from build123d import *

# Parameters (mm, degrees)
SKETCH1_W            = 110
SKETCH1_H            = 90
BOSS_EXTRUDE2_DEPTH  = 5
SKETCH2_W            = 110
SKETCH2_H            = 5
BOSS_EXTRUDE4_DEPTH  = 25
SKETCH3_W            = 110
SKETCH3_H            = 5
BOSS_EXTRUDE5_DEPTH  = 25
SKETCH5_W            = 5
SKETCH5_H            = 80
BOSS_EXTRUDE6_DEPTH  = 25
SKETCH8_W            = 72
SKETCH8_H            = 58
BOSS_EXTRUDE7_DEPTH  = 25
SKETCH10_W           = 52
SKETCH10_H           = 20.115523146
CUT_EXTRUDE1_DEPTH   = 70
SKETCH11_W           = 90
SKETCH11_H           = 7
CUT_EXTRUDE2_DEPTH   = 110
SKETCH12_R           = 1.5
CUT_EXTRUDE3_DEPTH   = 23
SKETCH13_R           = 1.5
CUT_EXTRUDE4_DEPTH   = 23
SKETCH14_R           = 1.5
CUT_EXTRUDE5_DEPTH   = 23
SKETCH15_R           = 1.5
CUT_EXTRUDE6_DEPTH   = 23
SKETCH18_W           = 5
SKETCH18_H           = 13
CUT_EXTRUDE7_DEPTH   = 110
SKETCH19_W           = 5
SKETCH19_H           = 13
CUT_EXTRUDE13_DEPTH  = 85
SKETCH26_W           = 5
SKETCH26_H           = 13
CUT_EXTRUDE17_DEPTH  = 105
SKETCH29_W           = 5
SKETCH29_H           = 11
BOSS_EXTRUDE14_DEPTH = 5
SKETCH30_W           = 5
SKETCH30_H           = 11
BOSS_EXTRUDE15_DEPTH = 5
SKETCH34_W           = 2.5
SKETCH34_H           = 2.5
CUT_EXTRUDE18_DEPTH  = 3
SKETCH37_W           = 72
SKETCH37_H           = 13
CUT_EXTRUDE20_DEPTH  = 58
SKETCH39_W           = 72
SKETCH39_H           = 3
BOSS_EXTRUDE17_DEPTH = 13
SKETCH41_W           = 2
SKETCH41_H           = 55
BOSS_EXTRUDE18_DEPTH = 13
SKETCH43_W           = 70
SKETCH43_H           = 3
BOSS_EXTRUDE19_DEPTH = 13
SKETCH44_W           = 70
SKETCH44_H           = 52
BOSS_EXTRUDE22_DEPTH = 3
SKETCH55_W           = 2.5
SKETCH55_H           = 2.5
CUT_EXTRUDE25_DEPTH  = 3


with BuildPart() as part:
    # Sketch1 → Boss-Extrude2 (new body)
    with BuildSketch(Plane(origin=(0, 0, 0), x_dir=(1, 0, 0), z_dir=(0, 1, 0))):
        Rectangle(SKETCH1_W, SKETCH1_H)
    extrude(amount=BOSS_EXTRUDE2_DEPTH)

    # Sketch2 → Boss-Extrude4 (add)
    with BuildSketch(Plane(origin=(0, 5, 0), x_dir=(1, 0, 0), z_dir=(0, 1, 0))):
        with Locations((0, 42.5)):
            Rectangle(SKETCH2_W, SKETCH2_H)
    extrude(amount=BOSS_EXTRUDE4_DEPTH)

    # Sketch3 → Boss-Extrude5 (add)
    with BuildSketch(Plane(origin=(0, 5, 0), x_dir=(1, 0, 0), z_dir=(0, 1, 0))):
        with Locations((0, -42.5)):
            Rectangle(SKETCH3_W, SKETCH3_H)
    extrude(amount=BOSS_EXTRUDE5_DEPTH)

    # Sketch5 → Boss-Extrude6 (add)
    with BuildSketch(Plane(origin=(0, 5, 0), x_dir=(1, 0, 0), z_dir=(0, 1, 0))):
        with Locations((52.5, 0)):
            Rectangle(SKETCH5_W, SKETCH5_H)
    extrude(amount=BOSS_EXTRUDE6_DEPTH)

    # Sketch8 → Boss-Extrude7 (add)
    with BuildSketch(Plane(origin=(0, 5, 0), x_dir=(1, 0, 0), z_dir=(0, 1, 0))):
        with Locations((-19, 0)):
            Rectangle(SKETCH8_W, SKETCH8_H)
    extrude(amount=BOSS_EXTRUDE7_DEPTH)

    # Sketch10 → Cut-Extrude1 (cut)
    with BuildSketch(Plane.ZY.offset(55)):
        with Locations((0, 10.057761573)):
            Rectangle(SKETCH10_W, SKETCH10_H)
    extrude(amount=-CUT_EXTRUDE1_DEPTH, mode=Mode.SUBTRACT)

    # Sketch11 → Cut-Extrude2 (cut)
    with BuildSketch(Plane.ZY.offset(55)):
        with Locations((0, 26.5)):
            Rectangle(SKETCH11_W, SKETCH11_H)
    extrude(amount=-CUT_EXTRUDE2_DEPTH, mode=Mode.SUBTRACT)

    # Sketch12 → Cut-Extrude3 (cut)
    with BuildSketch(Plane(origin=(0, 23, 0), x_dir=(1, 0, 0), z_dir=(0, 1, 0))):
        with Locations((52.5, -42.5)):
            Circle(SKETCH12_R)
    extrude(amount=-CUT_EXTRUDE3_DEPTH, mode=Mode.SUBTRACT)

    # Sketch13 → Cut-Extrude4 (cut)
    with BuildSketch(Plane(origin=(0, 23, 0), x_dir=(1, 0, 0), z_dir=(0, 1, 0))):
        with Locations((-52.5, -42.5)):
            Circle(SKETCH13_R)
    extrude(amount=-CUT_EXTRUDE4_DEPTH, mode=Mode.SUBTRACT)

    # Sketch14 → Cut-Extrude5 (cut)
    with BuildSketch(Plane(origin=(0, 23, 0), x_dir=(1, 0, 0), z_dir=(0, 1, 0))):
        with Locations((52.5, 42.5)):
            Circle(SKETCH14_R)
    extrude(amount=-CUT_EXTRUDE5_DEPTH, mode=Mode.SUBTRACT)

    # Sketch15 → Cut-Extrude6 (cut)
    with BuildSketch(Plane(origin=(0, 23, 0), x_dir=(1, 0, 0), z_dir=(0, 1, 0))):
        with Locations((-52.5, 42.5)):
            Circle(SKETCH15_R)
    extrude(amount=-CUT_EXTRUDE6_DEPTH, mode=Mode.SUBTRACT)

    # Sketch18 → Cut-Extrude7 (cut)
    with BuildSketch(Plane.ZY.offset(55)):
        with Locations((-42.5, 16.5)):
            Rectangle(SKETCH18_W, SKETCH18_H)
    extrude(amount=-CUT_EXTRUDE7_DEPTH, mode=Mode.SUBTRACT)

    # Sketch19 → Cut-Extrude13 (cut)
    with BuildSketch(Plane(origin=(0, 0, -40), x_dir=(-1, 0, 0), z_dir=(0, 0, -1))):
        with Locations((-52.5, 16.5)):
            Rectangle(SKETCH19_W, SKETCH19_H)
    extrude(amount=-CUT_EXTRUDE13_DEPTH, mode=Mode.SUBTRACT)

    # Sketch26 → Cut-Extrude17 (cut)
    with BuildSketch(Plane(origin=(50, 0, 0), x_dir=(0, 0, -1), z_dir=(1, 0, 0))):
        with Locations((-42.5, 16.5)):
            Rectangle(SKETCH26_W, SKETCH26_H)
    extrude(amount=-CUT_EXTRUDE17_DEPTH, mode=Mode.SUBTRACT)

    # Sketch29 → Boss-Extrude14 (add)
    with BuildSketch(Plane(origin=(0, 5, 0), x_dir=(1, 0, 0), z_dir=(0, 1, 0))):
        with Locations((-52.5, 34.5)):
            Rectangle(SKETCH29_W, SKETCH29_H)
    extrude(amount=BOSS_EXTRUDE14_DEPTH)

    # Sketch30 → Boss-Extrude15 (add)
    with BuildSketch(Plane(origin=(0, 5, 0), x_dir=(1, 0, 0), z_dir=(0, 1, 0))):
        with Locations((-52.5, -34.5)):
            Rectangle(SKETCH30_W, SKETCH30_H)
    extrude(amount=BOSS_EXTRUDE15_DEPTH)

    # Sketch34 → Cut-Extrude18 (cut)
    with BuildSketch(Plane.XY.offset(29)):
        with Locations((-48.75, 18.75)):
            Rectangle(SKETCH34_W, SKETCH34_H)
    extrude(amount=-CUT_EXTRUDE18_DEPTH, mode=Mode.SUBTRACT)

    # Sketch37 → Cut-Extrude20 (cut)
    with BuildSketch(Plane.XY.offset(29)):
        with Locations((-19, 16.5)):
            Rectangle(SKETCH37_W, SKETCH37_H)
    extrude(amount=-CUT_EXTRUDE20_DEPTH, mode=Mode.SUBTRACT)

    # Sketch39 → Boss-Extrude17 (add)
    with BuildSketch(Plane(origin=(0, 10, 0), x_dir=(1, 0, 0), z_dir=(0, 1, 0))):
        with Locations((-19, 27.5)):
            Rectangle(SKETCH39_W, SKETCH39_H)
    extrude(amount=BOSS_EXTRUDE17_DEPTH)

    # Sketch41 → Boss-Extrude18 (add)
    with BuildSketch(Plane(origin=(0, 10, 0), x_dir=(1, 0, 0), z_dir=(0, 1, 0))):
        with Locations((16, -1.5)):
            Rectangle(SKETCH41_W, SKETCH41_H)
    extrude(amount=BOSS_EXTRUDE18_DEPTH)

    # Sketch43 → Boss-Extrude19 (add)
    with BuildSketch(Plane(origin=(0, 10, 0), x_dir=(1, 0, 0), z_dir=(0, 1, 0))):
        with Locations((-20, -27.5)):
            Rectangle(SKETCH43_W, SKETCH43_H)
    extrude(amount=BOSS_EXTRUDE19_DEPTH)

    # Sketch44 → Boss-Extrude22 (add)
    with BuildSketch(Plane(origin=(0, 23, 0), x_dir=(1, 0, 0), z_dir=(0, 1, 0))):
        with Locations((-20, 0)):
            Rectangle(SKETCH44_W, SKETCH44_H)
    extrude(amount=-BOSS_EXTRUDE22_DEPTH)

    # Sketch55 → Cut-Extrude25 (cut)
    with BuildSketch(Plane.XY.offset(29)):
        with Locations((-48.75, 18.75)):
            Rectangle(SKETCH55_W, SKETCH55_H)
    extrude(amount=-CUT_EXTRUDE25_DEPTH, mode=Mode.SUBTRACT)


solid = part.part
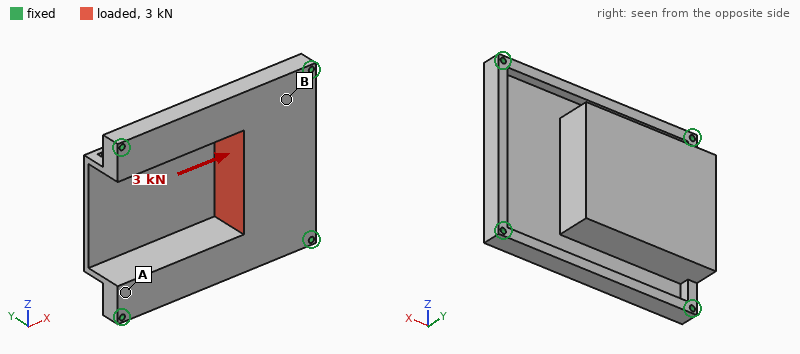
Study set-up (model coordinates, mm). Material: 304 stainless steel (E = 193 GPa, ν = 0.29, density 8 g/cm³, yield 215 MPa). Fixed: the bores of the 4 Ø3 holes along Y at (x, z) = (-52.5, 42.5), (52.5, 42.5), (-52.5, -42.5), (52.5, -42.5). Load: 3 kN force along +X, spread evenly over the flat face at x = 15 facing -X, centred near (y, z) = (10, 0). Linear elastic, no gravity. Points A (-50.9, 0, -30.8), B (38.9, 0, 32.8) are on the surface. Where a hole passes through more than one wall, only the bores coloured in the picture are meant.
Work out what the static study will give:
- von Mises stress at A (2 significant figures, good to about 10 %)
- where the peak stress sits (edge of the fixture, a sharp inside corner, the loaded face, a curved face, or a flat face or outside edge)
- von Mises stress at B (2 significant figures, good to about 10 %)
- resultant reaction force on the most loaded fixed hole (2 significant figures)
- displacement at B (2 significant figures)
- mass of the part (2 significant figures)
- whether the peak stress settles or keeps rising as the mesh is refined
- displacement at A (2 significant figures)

3.5 MPa
edge of the fixture
8.9 MPa
970 N
2.9 µm
480 g
keeps rising
1.2 µm
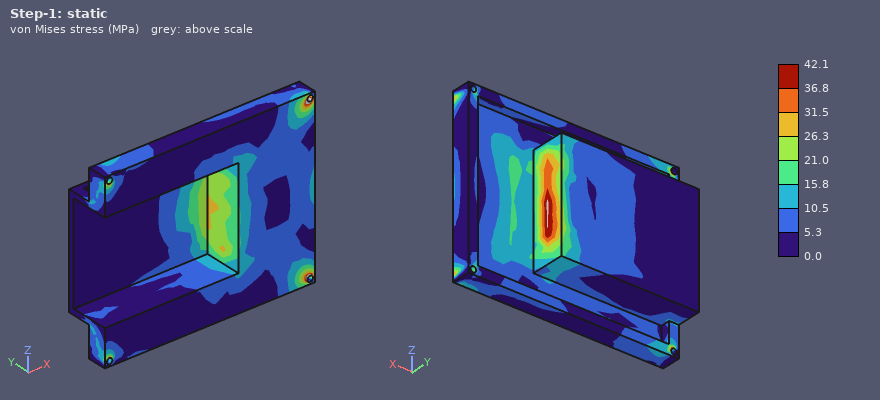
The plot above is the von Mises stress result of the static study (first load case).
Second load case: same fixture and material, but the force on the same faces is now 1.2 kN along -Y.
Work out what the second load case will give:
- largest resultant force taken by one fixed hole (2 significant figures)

430 N
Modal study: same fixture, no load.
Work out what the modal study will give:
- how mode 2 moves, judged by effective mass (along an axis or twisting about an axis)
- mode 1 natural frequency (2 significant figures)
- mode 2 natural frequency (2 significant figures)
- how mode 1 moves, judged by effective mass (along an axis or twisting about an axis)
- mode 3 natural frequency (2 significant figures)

along Z
2600 Hz
3600 Hz
along Y
4500 Hz
